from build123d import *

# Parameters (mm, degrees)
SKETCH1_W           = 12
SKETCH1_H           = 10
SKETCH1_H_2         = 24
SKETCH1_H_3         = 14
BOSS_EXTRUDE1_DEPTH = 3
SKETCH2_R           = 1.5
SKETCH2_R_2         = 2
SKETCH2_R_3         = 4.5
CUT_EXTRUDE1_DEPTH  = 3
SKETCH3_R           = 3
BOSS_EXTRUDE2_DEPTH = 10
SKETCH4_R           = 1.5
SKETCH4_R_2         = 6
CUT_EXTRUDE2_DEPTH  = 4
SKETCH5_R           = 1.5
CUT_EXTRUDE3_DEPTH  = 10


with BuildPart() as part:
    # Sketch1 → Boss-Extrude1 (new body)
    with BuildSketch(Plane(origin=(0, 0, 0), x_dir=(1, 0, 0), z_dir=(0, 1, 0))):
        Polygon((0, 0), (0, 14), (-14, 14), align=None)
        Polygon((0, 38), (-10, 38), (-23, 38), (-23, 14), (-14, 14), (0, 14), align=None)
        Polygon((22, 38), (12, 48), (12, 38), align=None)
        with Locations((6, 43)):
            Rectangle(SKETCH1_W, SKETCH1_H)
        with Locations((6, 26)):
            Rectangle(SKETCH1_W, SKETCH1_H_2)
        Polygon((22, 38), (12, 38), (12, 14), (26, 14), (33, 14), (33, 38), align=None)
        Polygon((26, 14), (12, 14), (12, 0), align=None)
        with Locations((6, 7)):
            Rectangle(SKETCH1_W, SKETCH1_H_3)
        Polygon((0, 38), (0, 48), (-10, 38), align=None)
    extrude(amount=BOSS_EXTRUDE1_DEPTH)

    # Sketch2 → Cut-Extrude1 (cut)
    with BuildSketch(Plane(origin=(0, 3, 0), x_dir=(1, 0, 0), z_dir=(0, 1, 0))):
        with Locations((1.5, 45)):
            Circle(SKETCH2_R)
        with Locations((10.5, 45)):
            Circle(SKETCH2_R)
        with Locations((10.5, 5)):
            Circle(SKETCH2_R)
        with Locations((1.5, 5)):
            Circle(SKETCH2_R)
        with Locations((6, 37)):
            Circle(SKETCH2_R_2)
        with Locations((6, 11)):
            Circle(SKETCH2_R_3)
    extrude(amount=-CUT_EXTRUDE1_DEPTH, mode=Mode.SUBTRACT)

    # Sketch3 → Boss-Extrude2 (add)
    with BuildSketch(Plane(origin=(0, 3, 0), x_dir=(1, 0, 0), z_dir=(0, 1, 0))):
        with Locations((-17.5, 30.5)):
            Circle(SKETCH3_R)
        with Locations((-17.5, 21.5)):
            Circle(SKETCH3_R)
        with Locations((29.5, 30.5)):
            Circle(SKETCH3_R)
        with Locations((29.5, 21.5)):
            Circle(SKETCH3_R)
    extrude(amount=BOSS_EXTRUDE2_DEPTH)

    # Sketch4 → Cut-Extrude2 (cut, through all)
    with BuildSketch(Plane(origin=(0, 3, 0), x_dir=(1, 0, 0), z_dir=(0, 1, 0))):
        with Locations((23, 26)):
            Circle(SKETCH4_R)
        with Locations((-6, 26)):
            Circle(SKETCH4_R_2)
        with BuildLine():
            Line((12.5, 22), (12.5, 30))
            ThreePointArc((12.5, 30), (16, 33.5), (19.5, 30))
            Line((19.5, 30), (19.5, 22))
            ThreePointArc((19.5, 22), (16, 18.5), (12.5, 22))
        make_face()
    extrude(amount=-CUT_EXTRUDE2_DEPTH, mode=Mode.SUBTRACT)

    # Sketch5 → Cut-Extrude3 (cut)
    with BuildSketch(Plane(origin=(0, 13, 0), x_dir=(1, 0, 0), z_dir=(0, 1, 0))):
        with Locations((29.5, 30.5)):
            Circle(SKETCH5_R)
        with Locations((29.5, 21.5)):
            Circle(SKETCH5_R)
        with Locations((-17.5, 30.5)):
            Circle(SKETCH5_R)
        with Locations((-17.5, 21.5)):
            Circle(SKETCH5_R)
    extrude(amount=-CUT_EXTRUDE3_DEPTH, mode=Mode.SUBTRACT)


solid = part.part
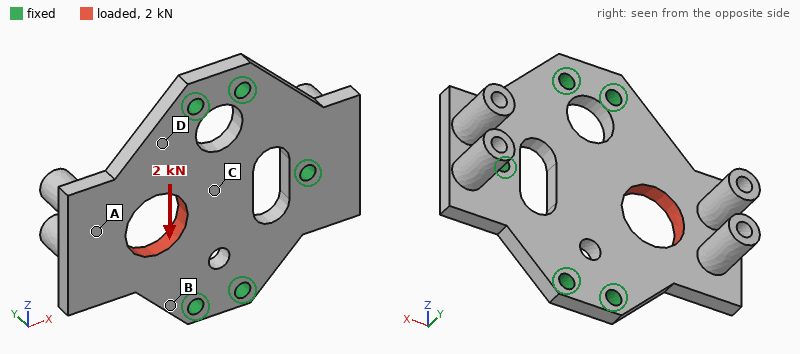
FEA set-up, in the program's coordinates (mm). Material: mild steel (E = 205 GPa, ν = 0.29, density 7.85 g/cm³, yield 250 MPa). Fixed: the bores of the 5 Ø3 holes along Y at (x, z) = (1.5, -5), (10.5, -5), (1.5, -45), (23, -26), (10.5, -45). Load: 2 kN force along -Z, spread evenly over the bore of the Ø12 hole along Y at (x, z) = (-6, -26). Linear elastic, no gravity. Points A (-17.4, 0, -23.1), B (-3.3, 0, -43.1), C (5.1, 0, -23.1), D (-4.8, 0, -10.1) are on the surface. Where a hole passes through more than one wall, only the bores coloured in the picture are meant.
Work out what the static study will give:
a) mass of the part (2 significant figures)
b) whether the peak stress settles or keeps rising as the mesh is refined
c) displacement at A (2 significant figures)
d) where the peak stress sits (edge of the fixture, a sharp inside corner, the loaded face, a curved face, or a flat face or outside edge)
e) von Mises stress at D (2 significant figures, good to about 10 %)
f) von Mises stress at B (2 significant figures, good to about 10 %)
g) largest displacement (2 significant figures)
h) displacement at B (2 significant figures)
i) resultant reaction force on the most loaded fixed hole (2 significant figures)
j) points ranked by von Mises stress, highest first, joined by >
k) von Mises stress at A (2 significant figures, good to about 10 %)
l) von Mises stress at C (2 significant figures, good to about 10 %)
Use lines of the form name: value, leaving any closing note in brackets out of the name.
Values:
mass of the part: 45 g
whether the peak stress settles or keeps rising as the mesh is refined: keeps rising
displacement at A: 4.0 µm
where the peak stress sits: edge of the fixture
von Mises stress at D: 28 MPa
von Mises stress at B: 37 MPa
largest displacement: 5.0 µm
displacement at B: 1.3 µm
resultant reaction force on the most loaded fixed hole: 880 N
points ranked by von Mises stress, highest first, joined by >: B > D > C > A
von Mises stress at A: 7.8 MPa
von Mises stress at C: 17 MPa
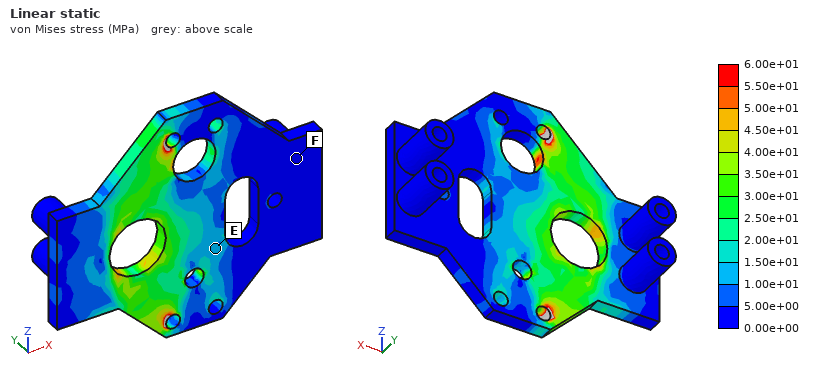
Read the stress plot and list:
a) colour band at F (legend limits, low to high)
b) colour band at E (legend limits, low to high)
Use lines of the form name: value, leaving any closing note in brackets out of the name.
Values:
colour band at F: 0.00e+00 to 5.00e+00 MPa
colour band at E: 1.00e+01 to 1.50e+01 MPa
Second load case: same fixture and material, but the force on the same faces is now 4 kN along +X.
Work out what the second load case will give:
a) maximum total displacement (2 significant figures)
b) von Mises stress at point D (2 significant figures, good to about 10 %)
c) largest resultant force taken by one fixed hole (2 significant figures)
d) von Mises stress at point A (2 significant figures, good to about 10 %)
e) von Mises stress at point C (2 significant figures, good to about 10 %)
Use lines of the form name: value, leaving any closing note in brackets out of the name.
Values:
maximum total displacement: 8.7 µm
von Mises stress at point D: 52 MPa
largest resultant force taken by one fixed hole: 1.1 kN
von Mises stress at point A: 32 MPa
von Mises stress at point C: 31 MPa
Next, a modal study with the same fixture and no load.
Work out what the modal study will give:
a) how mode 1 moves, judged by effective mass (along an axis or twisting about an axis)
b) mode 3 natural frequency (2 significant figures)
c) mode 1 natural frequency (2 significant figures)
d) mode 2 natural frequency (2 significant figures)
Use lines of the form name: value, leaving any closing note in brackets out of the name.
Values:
how mode 1 moves, judged by effective mass: along Y
mode 3 natural frequency: 9600 Hz
mode 1 natural frequency: 2700 Hz
mode 2 natural frequency: 7800 Hz
